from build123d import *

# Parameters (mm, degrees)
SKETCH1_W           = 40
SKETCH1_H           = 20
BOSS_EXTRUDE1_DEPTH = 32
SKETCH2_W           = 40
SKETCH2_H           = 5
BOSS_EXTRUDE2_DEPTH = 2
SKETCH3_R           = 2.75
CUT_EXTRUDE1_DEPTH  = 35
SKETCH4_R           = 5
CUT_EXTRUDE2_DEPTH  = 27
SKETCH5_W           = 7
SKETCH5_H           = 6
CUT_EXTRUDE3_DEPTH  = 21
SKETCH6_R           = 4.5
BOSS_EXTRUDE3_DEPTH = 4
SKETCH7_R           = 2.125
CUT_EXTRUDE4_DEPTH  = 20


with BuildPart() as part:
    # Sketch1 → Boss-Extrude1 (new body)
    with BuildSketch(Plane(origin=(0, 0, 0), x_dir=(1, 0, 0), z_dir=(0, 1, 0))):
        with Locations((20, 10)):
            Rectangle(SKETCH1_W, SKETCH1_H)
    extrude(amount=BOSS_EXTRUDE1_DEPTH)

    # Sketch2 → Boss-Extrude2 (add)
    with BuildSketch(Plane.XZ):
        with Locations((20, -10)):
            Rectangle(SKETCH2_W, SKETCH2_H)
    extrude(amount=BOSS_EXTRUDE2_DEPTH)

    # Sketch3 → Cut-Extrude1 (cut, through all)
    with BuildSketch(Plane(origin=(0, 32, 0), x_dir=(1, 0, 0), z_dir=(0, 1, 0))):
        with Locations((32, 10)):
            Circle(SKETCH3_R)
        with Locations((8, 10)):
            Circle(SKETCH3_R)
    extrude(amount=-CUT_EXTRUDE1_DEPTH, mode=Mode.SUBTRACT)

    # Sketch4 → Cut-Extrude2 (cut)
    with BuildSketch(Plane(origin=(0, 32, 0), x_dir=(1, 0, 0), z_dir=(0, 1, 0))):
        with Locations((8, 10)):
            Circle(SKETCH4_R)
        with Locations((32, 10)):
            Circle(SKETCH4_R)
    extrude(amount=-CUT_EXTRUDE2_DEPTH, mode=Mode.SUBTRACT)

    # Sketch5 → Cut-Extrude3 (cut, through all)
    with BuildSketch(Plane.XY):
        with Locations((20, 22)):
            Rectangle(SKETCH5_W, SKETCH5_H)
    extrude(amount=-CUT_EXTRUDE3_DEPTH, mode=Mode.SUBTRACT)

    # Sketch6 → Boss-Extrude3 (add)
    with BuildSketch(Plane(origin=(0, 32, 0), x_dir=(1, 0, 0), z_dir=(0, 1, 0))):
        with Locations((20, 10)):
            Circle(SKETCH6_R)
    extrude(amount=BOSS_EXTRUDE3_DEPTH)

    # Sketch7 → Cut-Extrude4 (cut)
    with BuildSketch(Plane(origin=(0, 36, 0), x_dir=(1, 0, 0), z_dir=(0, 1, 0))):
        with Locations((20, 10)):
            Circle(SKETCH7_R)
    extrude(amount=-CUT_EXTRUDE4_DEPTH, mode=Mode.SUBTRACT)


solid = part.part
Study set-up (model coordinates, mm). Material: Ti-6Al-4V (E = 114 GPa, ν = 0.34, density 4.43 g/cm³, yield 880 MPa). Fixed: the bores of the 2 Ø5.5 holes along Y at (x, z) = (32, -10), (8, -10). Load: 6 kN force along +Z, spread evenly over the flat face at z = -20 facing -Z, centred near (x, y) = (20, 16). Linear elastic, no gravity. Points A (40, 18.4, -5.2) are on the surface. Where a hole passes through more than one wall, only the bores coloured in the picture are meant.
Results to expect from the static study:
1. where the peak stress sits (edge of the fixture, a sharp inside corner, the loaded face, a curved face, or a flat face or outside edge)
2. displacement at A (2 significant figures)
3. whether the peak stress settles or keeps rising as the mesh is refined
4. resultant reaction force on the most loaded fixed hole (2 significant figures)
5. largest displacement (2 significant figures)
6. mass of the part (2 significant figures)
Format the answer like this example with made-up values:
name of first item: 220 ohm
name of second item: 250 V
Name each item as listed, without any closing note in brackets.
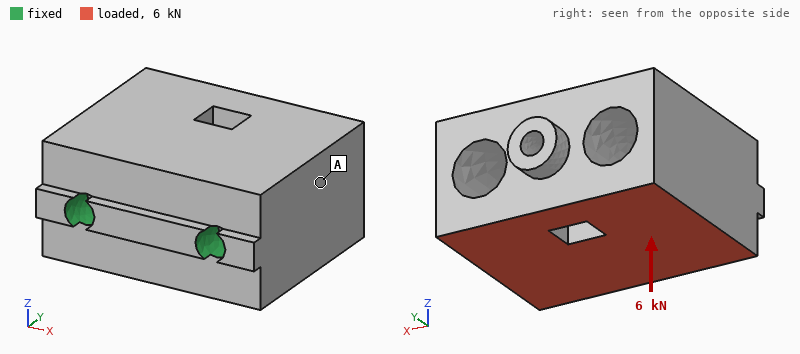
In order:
where the peak stress sits: edge of the fixture
displacement at A: 43 µm
whether the peak stress settles or keeps rising as the mesh is refined: keeps rising
resultant reaction force on the most loaded fixed hole: 3.0 kN
largest displacement: 87 µm
mass of the part: 91 g
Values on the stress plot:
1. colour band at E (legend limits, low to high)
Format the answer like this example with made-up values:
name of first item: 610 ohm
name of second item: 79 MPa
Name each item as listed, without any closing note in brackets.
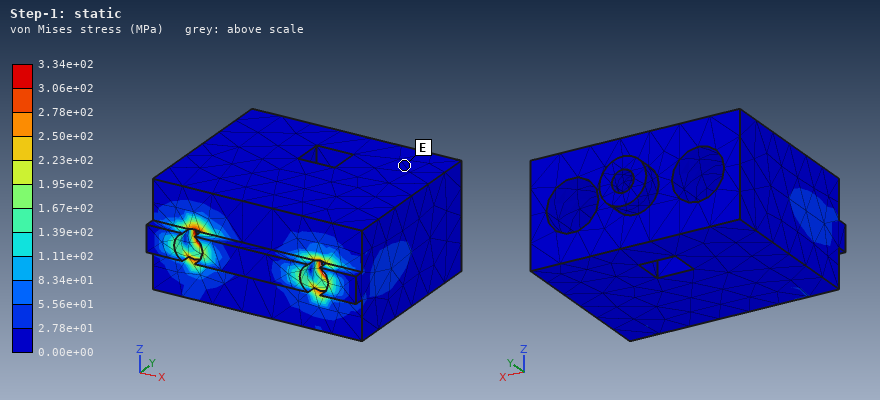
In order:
colour band at E: 0.00e+00 to 2.78e+01 MPa
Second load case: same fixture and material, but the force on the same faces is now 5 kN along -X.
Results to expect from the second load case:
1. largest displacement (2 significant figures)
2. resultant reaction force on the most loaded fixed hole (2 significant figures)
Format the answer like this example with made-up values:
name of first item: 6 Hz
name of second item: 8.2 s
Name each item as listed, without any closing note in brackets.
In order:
largest displacement: 18 µm
resultant reaction force on the most loaded fixed hole: 3.9 kN
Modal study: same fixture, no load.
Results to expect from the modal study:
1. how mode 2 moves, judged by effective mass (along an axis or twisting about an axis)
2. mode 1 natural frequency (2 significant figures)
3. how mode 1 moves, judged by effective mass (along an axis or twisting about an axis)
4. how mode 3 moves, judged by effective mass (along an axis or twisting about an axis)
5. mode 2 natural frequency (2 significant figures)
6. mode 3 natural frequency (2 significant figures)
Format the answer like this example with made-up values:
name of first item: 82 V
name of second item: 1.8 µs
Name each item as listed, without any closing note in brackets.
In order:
how mode 2 moves, judged by effective mass: along X
mode 1 natural frequency: 5400 Hz
how mode 1 moves, judged by effective mass: along Z
how mode 3 moves, judged by effective mass: twisting about Y
mode 2 natural frequency: 12 kHz
mode 3 natural frequency: 16 kHz
